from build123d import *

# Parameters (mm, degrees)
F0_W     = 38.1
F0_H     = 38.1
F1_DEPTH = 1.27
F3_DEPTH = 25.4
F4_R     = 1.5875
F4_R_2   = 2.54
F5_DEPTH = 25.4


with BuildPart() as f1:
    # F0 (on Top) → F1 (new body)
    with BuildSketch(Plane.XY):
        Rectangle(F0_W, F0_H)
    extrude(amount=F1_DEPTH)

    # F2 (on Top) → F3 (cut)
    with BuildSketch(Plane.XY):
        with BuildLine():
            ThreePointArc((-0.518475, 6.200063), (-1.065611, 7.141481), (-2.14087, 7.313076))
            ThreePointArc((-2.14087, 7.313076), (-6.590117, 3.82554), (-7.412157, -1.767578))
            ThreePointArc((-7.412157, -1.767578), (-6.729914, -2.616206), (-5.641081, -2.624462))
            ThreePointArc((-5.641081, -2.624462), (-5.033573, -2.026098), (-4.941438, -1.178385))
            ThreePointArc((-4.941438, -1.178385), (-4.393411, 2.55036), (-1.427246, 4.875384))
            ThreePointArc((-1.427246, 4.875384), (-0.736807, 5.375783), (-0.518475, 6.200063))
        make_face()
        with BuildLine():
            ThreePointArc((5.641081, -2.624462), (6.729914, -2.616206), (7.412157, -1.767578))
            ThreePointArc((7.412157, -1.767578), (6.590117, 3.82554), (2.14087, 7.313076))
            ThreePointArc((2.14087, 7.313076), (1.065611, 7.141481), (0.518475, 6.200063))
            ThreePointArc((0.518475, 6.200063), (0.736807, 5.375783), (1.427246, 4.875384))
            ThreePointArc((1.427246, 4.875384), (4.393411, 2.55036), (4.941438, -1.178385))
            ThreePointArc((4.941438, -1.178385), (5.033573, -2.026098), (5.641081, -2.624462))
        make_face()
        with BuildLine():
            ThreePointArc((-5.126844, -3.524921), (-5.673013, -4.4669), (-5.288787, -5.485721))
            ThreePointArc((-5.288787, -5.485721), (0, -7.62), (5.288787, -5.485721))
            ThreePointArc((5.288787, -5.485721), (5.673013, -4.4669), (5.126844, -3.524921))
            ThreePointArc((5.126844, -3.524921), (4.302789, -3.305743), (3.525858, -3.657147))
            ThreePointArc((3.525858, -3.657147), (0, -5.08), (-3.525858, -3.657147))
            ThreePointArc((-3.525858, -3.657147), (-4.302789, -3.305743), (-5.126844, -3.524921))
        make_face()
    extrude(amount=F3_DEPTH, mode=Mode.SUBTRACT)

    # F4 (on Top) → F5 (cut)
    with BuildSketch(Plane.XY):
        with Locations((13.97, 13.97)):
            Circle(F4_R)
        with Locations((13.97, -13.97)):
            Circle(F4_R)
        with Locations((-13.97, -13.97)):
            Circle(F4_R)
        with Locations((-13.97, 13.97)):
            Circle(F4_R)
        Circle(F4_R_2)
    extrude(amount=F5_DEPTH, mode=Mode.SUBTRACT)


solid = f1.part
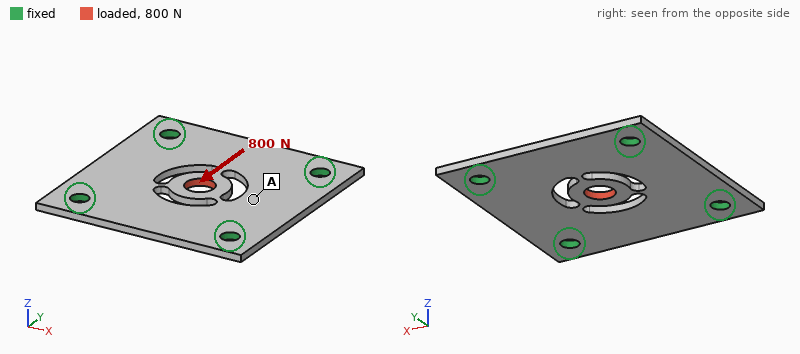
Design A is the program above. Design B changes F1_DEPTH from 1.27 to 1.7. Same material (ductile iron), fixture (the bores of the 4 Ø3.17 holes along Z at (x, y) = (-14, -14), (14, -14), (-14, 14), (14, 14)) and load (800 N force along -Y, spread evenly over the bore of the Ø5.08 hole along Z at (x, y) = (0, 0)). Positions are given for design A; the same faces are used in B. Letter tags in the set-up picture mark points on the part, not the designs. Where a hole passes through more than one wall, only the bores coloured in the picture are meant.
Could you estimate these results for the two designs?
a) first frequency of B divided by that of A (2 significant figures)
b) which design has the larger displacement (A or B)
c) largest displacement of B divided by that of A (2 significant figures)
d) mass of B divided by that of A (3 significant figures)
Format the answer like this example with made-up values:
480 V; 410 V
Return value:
1.3; A; 0.75; 1.34
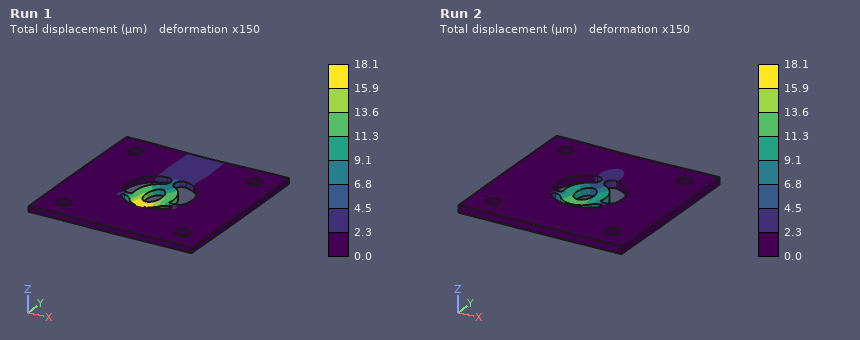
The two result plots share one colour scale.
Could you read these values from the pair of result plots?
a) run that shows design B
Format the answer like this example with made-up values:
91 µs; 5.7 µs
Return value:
Run 2
